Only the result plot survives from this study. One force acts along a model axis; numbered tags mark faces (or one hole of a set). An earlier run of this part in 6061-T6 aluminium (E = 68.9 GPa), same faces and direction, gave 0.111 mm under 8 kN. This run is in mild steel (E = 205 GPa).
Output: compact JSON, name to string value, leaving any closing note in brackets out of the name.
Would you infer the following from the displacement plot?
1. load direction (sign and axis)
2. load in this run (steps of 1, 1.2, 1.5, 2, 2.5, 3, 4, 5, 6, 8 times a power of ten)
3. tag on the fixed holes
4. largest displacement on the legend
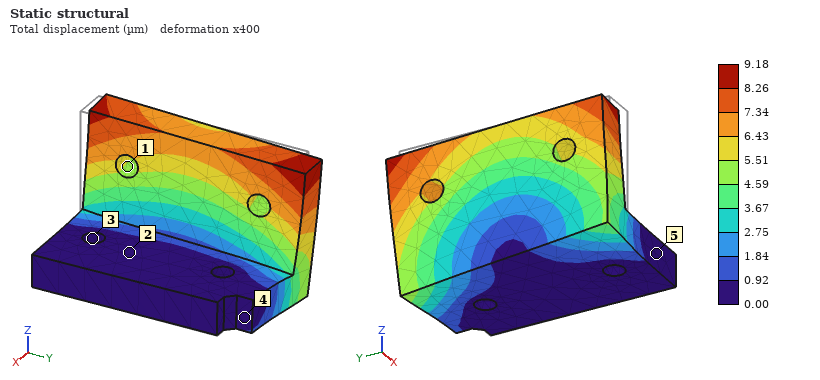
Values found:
{"load direction": "+Y", "load in this run": "2 kN", "tag on the fixed holes": "3", "largest displacement on the legend": "9.18 µm"}
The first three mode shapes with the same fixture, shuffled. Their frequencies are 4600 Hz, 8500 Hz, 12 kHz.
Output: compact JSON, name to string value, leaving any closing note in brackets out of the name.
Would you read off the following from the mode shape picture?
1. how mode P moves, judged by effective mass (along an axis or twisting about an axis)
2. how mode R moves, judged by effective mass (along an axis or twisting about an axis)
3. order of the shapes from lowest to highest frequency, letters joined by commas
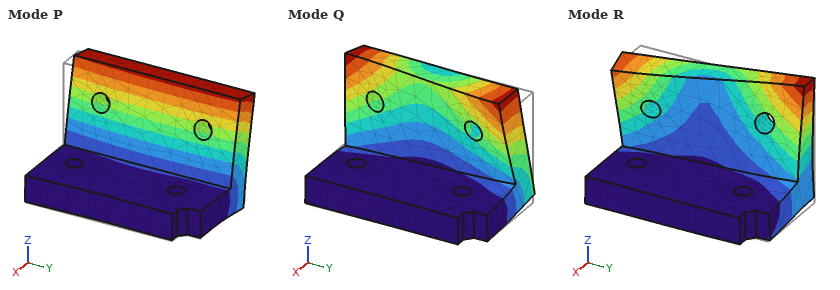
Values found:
{"how mode P moves, judged by effective mass": "along X", "how mode R moves, judged by effective mass": "along Y", "order of the shapes from lowest to highest frequency, letters joined by commas": "P, Q, R"}
